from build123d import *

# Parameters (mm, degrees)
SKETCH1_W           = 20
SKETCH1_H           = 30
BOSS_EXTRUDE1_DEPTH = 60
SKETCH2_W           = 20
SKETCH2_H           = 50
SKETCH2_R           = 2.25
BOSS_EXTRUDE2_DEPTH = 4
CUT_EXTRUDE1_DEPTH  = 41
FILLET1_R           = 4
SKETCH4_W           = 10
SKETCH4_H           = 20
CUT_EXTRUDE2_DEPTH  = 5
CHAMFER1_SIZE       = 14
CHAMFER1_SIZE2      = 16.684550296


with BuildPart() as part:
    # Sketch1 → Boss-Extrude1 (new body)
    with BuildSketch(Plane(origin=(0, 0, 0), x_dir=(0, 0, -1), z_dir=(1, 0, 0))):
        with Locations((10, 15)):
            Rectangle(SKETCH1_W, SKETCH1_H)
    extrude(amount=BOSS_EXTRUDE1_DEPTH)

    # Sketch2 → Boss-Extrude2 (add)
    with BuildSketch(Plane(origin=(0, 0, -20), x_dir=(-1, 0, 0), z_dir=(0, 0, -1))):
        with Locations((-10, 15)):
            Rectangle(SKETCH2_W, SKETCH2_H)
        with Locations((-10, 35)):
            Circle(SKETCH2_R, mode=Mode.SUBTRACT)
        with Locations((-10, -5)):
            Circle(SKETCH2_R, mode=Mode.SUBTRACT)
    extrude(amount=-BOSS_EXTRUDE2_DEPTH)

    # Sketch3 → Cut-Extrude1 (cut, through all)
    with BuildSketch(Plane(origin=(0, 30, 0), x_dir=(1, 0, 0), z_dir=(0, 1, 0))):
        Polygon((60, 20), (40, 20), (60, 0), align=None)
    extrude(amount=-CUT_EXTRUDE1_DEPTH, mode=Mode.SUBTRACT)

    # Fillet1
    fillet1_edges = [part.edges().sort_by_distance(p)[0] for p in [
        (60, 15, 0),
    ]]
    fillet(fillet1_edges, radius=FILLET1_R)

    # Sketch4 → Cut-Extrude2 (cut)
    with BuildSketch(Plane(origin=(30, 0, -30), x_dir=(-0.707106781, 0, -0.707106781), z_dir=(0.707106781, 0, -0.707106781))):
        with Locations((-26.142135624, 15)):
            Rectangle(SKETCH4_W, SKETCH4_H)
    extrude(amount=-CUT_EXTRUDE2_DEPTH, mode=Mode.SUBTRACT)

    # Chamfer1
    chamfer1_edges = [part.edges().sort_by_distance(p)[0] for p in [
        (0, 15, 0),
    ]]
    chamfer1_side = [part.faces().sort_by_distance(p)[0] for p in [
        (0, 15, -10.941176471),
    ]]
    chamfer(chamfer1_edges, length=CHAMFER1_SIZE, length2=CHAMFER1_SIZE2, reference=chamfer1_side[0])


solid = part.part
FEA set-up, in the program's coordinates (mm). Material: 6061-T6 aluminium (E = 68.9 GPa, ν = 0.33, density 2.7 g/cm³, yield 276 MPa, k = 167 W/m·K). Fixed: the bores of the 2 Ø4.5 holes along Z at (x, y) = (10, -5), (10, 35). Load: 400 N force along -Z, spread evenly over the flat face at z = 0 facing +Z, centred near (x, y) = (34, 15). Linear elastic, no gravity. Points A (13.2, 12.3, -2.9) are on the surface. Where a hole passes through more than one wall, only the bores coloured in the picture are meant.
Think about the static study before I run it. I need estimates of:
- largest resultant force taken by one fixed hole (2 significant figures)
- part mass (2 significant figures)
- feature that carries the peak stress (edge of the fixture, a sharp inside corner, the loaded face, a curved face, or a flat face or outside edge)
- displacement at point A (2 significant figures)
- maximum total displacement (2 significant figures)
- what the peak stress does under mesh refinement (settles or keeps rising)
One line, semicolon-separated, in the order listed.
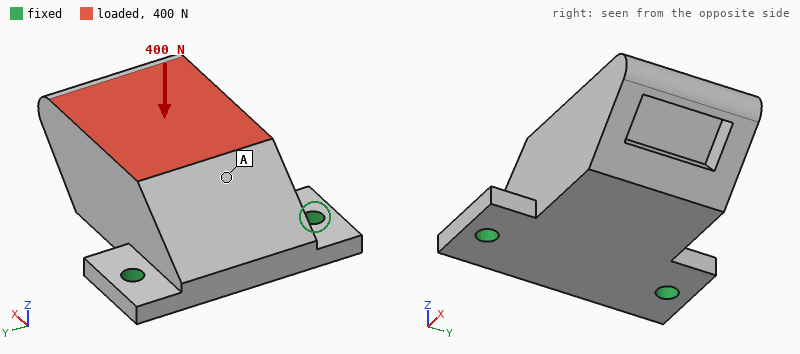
220 N; 71 g; edge of the fixture; 0.035 mm; 0.11 mm; keeps rising
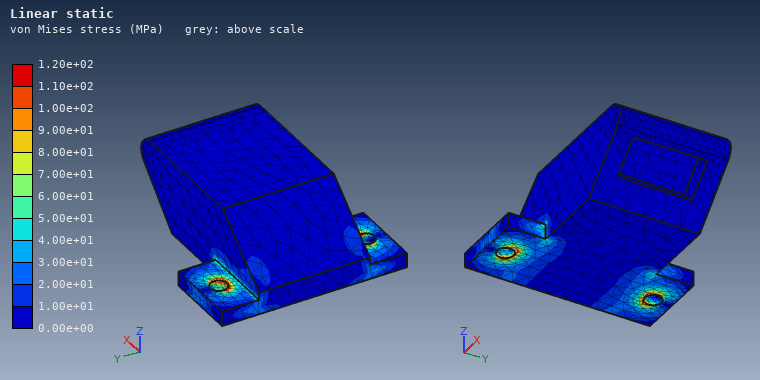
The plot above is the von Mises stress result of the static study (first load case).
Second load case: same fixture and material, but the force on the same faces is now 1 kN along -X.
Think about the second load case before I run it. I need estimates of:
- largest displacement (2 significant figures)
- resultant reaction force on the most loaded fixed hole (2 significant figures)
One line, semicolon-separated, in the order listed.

0.21 mm; 500 N
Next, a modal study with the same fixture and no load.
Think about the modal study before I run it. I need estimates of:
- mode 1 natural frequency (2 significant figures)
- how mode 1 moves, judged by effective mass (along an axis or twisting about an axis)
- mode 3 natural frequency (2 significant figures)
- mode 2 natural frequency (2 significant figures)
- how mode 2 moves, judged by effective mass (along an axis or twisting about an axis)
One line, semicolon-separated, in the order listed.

1700 Hz; along Z; 11 kHz; 7700 Hz; along Y
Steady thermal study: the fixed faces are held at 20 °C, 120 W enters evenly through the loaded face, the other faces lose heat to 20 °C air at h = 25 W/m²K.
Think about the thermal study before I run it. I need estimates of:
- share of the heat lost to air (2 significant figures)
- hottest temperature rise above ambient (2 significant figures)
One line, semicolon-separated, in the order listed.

5.5 %; 73 K
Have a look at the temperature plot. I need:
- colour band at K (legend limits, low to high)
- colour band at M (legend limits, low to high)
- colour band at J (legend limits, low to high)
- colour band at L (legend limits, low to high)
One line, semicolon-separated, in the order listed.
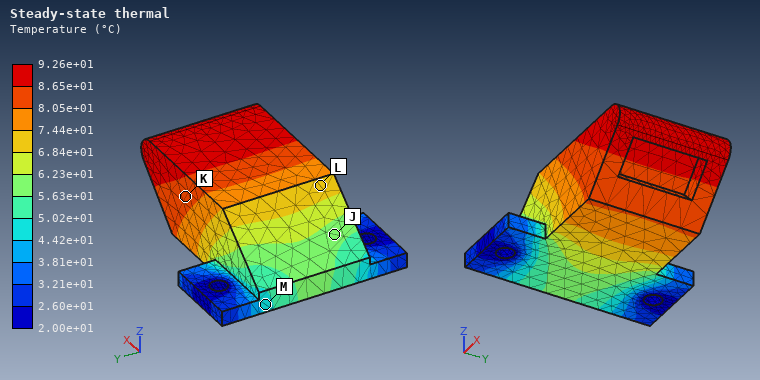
8.05e+01 to 8.65e+01 °C; 4.42e+01 to 5.02e+01 °C; 5.63e+01 to 6.23e+01 °C; 6.84e+01 to 7.44e+01 °C
